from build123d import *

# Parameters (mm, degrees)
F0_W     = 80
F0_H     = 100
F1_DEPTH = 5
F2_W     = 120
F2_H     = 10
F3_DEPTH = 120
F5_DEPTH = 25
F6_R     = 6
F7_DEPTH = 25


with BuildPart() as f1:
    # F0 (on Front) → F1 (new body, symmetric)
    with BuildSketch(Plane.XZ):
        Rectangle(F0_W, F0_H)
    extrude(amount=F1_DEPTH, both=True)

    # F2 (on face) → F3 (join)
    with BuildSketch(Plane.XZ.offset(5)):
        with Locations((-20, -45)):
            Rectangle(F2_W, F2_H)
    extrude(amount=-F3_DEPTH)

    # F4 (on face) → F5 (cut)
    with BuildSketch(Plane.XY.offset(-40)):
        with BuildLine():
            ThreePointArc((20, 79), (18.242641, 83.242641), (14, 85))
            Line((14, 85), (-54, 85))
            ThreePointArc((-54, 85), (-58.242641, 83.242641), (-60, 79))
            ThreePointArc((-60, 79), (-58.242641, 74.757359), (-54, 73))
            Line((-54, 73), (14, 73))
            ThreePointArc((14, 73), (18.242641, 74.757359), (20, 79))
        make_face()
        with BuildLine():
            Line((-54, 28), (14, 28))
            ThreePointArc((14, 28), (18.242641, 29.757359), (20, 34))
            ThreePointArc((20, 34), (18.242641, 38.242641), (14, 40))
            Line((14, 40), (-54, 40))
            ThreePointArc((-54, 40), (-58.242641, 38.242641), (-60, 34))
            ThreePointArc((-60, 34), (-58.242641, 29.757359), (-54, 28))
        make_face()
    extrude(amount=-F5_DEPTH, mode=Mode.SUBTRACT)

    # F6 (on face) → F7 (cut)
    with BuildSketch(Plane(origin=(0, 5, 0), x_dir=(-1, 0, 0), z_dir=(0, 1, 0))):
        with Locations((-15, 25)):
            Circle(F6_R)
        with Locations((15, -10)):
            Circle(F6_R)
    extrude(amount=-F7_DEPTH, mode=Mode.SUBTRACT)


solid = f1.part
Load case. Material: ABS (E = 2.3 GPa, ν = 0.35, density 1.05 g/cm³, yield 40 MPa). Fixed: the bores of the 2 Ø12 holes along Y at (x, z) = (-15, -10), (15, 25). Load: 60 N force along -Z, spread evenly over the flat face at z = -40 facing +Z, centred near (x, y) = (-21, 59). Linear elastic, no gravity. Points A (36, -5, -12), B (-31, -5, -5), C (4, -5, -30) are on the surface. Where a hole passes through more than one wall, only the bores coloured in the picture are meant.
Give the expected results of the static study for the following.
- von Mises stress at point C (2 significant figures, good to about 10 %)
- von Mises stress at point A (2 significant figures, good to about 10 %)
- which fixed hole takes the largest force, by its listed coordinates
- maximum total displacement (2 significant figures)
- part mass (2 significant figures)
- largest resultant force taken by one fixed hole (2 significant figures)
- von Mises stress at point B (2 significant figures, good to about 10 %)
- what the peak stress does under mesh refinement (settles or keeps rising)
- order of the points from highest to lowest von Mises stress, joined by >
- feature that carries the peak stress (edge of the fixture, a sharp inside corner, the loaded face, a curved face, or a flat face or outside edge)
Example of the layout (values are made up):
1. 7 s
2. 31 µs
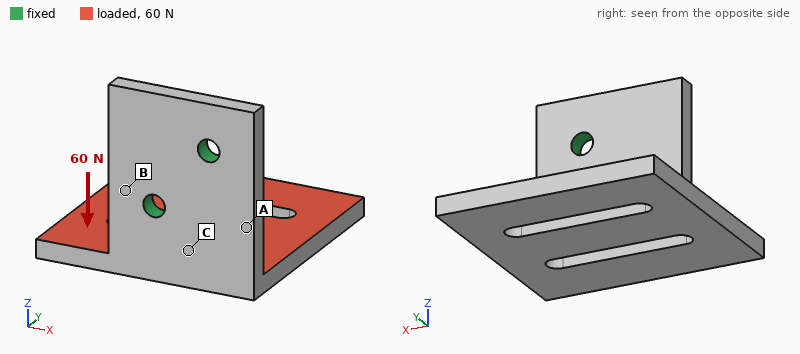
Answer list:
1. 2.2 MPa
2. 1.5 MPa
3. (-15, -10)
4. 2.2 mm
5. 200 g
6. 67 N
7. 0.52 MPa
8. keeps rising
9. C > A > B
10. edge of the fixture
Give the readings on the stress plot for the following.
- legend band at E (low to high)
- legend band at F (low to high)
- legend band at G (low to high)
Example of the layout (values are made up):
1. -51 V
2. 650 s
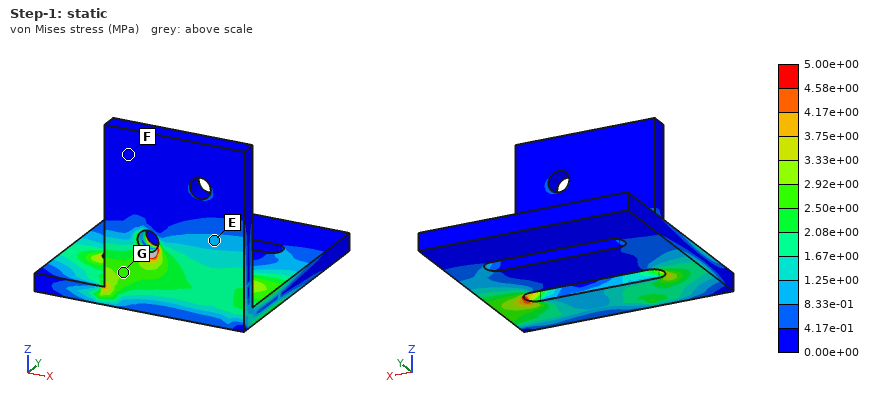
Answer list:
1. 8.33e-01 to 1.25e+00 MPa
2. 0.00e+00 to 4.17e-01 MPa
3. 2.50e+00 to 2.92e+00 MPa
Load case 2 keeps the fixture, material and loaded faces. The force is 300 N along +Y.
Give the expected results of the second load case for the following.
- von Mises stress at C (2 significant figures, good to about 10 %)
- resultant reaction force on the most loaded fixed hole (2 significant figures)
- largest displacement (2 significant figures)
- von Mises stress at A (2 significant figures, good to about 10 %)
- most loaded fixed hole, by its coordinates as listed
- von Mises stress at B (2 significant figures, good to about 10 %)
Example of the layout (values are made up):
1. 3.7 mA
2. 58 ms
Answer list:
1. 2.7 MPa
2. 350 N
3. 0.82 mm
4. 1.4 MPa
5. (-15, -10)
6. 2.5 MPa
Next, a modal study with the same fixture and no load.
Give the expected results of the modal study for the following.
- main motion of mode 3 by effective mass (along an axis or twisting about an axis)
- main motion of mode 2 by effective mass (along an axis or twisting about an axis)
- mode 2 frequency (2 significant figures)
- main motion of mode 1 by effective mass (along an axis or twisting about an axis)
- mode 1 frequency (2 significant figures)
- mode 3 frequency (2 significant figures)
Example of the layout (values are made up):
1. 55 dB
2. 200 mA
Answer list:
1. twisting about Y
2. along X
3. 160 Hz
4. along Z
5. 94 Hz
6. 300 Hz
